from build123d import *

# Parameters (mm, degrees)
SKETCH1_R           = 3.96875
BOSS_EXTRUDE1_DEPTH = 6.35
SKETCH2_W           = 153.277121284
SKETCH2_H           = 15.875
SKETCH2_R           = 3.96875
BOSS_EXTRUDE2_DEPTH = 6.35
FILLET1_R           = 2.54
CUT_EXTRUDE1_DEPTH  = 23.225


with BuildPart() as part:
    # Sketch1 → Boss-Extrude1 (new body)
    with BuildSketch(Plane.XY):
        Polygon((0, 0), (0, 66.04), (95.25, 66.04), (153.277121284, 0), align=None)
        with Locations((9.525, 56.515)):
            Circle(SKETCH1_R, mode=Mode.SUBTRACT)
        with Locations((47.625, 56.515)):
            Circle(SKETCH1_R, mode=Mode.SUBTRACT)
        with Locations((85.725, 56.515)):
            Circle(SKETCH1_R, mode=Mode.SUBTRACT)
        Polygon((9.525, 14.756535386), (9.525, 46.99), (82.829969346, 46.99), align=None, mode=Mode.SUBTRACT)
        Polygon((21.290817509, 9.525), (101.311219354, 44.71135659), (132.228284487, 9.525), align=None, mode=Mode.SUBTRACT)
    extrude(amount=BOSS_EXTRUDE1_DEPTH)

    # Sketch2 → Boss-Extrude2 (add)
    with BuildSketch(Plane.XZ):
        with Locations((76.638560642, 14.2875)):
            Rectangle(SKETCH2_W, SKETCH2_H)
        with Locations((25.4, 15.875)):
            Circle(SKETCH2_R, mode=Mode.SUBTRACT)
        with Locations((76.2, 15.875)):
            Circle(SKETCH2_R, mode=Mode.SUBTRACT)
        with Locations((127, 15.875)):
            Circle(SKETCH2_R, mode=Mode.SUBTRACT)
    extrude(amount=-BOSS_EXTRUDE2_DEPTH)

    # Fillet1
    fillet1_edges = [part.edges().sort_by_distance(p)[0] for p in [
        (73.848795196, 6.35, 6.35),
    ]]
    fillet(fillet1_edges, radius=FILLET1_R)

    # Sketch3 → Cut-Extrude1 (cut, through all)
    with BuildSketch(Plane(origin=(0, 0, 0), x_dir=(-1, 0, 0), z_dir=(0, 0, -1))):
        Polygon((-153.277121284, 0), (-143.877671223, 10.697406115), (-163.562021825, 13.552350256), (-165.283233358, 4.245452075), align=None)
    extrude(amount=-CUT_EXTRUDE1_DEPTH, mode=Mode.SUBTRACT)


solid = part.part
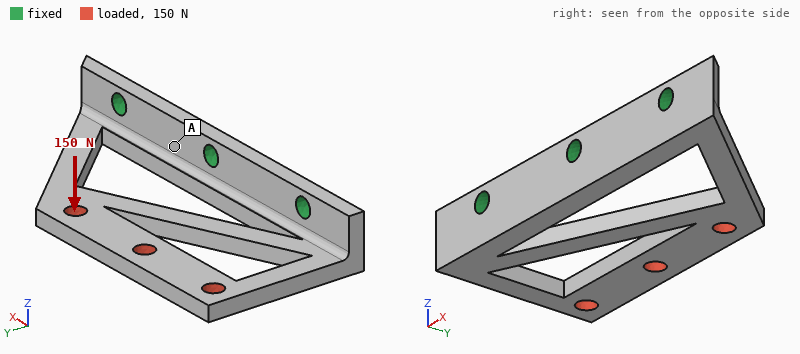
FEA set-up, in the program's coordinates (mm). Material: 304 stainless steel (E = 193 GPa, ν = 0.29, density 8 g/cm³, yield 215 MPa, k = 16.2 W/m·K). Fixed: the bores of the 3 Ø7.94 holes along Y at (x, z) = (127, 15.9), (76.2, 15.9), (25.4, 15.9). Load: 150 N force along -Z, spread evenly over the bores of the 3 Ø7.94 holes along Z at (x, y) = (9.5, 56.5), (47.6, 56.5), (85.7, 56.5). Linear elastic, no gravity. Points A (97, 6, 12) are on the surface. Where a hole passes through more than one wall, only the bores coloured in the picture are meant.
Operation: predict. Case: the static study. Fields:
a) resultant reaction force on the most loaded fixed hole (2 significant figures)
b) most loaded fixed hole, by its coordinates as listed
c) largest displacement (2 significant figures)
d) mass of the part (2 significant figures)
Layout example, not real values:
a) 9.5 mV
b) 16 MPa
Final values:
a) 120 N
b) (25.4, 15.9)
c) 0.13 mm
d) 370 g
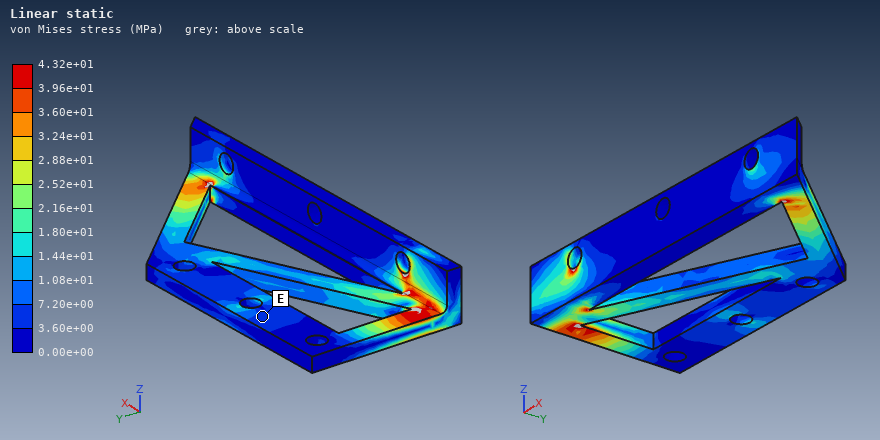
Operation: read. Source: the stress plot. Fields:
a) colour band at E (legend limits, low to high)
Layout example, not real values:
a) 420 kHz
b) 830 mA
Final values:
a) 3.60e+00 to 7.20e+00 MPa
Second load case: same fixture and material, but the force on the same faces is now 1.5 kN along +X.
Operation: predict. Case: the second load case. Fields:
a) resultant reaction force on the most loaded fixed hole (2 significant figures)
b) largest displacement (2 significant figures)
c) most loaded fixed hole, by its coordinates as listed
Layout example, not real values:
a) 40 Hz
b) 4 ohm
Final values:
a) 960 N
b) 36 µm
c) (25.4, 15.9)
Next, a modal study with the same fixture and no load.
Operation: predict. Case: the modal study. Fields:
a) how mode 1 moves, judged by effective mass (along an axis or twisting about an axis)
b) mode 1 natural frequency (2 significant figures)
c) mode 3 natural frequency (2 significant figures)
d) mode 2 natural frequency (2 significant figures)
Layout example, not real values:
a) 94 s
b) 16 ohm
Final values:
a) along Z
b) 580 Hz
c) 2800 Hz
d) 1400 Hz
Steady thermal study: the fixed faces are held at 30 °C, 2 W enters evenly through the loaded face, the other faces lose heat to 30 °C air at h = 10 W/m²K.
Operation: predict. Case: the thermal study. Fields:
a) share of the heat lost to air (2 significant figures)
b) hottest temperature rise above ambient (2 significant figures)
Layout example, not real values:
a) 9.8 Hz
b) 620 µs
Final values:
a) 72 %
b) 22 K
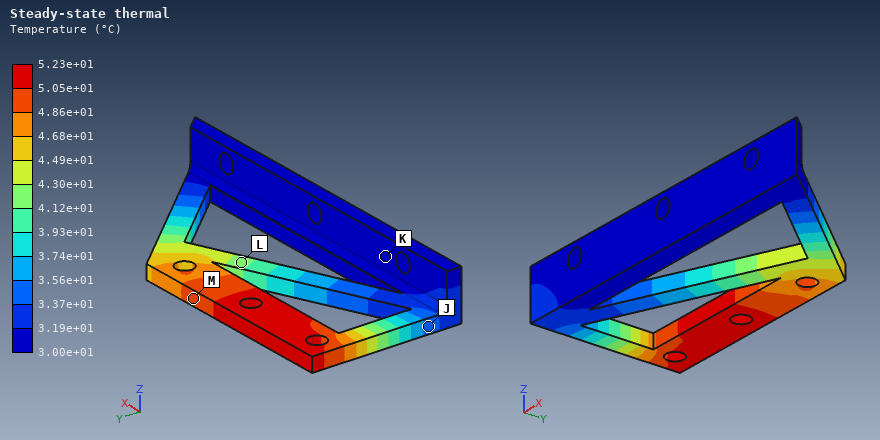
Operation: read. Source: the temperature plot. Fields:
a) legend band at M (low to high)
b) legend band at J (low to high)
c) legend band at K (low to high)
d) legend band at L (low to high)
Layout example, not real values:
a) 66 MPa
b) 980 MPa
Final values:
a) 4.86e+01 to 5.05e+01 °C
b) 3.37e+01 to 3.56e+01 °C
c) 3.00e+01 to 3.19e+01 °C
d) 4.12e+01 to 4.30e+01 °C
